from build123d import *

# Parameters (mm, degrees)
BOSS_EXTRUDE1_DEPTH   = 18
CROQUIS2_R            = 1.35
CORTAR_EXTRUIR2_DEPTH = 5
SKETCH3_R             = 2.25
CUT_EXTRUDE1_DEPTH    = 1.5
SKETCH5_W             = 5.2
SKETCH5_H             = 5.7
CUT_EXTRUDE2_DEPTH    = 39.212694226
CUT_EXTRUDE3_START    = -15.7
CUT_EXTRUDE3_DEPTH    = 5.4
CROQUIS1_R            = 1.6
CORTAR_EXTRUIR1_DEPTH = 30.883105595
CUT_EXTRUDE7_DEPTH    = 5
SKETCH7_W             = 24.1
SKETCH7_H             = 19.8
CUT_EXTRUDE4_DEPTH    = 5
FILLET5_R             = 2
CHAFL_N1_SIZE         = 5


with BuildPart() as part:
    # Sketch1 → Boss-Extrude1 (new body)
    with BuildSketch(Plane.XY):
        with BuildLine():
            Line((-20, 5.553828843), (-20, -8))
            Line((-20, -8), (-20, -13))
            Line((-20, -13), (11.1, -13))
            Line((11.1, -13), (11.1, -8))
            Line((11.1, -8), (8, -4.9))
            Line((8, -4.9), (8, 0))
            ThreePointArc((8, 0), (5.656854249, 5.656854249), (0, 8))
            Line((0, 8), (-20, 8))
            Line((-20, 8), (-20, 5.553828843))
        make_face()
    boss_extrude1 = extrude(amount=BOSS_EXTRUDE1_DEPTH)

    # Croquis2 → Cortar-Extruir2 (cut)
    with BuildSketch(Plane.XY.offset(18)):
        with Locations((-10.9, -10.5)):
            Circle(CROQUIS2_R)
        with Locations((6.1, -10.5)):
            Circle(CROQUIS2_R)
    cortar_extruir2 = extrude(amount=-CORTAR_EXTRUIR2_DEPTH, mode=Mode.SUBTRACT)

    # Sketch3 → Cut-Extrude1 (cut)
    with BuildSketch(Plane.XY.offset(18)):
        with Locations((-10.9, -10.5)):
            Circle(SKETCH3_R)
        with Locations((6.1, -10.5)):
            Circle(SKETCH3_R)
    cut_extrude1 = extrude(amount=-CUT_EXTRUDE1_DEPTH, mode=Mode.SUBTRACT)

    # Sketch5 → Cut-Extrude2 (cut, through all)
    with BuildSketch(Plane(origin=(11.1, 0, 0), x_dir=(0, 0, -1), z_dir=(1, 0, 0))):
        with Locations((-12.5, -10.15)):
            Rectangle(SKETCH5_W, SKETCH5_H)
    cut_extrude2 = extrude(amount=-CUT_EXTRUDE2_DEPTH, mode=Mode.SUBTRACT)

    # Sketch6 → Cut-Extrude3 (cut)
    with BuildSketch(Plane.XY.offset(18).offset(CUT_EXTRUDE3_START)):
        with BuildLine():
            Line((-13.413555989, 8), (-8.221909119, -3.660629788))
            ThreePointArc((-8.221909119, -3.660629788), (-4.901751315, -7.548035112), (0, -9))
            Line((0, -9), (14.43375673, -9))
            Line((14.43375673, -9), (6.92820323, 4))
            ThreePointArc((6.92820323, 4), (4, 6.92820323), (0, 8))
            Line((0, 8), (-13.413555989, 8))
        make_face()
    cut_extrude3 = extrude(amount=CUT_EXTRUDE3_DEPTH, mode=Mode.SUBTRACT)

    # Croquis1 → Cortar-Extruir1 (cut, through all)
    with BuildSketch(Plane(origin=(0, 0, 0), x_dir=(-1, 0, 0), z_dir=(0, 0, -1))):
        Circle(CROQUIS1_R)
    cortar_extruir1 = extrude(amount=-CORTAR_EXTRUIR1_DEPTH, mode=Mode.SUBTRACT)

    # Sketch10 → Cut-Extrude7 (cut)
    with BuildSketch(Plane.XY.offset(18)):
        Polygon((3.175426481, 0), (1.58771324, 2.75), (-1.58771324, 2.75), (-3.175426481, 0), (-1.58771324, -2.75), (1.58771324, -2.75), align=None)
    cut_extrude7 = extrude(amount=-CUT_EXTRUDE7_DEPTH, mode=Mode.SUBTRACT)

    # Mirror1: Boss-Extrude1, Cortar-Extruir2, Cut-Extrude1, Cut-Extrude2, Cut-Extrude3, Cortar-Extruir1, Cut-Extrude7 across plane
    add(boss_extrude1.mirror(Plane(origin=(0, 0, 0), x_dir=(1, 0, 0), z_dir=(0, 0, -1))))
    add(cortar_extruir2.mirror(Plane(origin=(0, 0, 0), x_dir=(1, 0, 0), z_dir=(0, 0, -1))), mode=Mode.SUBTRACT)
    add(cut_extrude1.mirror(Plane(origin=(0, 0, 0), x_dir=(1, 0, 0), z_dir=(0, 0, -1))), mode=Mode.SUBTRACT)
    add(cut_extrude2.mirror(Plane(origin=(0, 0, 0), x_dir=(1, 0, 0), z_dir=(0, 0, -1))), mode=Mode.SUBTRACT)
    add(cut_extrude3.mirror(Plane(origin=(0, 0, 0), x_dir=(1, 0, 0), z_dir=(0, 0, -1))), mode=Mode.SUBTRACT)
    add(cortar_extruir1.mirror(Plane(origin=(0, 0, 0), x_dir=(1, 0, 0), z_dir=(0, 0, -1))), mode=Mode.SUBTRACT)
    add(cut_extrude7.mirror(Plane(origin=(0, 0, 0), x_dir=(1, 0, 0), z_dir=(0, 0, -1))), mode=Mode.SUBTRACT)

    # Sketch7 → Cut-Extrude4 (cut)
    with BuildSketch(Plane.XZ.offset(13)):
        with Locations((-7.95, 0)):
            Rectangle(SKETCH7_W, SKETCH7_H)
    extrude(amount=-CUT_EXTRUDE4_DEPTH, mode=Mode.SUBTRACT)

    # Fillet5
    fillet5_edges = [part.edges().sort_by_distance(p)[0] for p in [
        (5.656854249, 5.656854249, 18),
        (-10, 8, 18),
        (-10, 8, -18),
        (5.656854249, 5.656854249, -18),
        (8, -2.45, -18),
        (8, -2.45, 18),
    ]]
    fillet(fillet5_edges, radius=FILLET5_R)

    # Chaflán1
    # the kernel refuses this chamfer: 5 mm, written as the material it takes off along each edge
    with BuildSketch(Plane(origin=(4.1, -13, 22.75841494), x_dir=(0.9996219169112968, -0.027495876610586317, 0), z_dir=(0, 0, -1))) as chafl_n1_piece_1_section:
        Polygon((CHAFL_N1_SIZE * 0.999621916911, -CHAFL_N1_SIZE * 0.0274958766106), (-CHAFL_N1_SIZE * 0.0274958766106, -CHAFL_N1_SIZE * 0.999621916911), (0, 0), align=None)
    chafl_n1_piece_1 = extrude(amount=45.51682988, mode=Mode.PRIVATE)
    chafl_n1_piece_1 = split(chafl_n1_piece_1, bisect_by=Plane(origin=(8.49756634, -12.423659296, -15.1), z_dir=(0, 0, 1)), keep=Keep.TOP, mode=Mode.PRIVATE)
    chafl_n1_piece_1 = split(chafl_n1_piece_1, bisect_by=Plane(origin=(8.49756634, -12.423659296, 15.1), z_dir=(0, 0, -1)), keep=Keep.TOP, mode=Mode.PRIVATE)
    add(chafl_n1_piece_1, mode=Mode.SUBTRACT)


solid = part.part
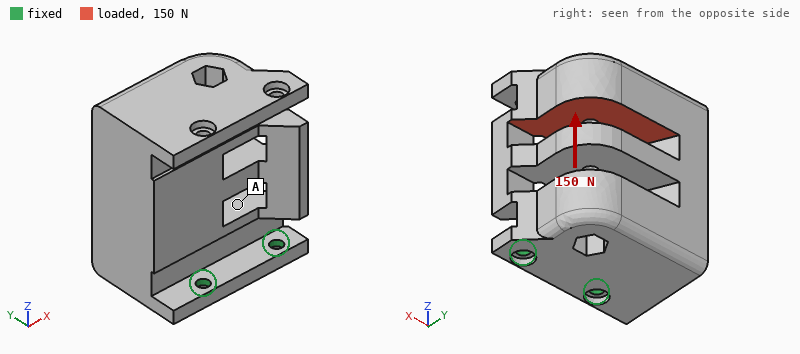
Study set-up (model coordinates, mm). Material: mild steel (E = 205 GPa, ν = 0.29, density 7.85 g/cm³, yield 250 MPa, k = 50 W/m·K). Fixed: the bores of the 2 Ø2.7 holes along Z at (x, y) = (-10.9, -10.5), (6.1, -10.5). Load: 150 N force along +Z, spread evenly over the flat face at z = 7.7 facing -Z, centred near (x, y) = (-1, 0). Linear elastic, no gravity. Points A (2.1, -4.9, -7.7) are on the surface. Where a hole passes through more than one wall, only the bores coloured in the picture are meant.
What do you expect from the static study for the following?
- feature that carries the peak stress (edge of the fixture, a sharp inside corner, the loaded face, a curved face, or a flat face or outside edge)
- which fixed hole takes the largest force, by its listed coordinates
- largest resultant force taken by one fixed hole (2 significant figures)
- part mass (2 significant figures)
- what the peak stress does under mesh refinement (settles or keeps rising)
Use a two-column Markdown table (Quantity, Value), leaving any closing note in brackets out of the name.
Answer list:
| Quantity | Value |
|---|---|
| feature that carries the peak stress | edge of the fixture |
| which fixed hole takes the largest force, by its listed coordinates | (6.1, -10.5) |
| largest resultant force taken by one fixed hole | 88 N |
| part mass | 100 g |
| what the peak stress does under mesh refinement | keeps rising |
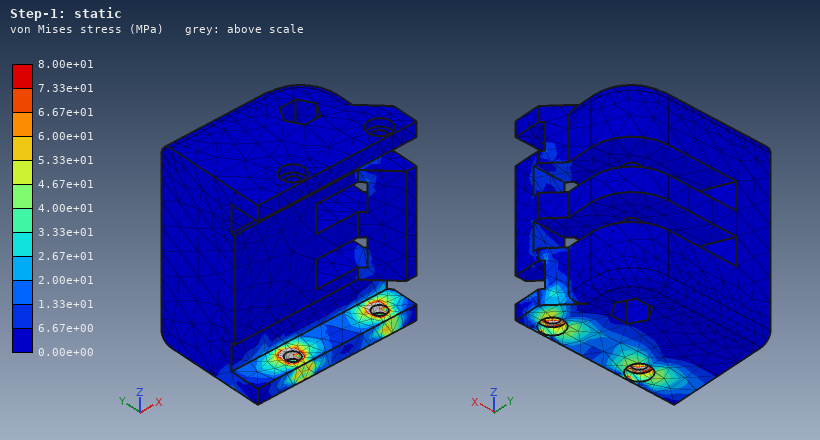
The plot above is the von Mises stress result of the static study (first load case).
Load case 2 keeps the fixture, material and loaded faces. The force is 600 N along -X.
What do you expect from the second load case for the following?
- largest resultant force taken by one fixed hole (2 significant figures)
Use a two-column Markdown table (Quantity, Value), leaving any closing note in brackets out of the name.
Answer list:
| Quantity | Value |
|---|---|
| largest resultant force taken by one fixed hole | 900 N |
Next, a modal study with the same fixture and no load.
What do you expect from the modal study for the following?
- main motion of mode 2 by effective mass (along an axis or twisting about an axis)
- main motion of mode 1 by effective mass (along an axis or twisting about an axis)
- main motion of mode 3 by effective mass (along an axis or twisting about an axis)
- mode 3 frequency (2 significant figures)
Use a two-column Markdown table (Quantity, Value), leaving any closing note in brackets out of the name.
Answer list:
| Quantity | Value |
|---|---|
| main motion of mode 2 by effective mass | along X |
| main motion of mode 1 by effective mass | along Y |
| main motion of mode 3 by effective mass | along Z |
| mode 3 frequency | 6700 Hz |
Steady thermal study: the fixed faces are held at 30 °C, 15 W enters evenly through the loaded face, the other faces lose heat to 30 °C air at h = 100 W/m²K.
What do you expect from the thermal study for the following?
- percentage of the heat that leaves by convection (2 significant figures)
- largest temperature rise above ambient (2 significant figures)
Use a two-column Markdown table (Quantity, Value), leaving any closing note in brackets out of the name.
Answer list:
| Quantity | Value |
|---|---|
| percentage of the heat that leaves by convection | 75 % |
| largest temperature rise above ambient | 42 K |
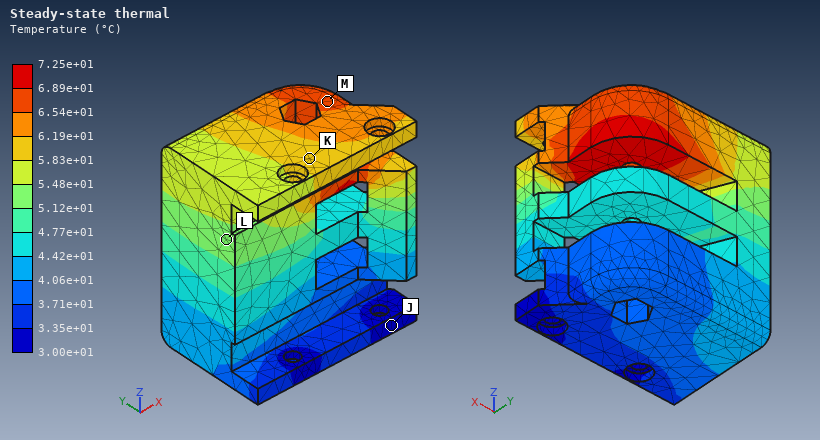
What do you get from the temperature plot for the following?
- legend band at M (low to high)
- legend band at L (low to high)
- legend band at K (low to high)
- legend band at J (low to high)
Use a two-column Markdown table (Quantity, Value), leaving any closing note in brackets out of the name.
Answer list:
| Quantity | Value |
|---|---|
| legend band at M | 6.54e+01 to 6.89e+01 °C |
| legend band at L | 5.12e+01 to 5.48e+01 °C |
| legend band at K | 5.83e+01 to 6.19e+01 °C |
| legend band at J | 3.00e+01 to 3.35e+01 °C |
